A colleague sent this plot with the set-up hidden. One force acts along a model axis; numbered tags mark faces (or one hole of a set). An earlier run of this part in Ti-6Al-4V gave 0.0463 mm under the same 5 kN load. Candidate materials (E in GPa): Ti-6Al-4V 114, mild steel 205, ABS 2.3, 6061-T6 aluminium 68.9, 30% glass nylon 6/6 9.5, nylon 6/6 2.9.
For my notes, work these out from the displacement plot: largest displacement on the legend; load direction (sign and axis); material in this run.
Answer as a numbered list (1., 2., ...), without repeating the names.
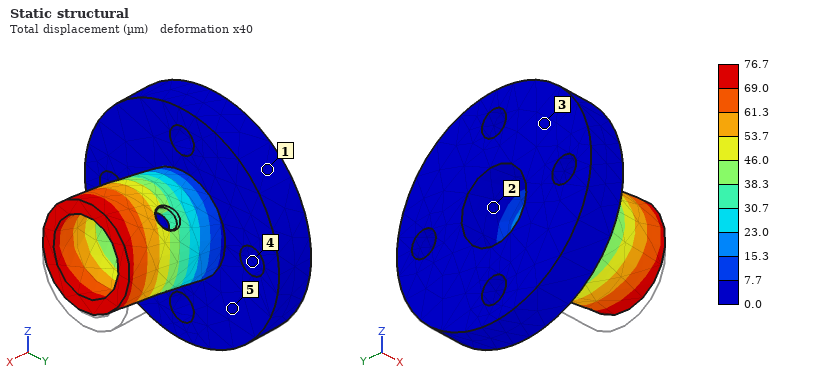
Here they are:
1. 76.7 µm
2. +Z
3. 6061-T6 aluminium
